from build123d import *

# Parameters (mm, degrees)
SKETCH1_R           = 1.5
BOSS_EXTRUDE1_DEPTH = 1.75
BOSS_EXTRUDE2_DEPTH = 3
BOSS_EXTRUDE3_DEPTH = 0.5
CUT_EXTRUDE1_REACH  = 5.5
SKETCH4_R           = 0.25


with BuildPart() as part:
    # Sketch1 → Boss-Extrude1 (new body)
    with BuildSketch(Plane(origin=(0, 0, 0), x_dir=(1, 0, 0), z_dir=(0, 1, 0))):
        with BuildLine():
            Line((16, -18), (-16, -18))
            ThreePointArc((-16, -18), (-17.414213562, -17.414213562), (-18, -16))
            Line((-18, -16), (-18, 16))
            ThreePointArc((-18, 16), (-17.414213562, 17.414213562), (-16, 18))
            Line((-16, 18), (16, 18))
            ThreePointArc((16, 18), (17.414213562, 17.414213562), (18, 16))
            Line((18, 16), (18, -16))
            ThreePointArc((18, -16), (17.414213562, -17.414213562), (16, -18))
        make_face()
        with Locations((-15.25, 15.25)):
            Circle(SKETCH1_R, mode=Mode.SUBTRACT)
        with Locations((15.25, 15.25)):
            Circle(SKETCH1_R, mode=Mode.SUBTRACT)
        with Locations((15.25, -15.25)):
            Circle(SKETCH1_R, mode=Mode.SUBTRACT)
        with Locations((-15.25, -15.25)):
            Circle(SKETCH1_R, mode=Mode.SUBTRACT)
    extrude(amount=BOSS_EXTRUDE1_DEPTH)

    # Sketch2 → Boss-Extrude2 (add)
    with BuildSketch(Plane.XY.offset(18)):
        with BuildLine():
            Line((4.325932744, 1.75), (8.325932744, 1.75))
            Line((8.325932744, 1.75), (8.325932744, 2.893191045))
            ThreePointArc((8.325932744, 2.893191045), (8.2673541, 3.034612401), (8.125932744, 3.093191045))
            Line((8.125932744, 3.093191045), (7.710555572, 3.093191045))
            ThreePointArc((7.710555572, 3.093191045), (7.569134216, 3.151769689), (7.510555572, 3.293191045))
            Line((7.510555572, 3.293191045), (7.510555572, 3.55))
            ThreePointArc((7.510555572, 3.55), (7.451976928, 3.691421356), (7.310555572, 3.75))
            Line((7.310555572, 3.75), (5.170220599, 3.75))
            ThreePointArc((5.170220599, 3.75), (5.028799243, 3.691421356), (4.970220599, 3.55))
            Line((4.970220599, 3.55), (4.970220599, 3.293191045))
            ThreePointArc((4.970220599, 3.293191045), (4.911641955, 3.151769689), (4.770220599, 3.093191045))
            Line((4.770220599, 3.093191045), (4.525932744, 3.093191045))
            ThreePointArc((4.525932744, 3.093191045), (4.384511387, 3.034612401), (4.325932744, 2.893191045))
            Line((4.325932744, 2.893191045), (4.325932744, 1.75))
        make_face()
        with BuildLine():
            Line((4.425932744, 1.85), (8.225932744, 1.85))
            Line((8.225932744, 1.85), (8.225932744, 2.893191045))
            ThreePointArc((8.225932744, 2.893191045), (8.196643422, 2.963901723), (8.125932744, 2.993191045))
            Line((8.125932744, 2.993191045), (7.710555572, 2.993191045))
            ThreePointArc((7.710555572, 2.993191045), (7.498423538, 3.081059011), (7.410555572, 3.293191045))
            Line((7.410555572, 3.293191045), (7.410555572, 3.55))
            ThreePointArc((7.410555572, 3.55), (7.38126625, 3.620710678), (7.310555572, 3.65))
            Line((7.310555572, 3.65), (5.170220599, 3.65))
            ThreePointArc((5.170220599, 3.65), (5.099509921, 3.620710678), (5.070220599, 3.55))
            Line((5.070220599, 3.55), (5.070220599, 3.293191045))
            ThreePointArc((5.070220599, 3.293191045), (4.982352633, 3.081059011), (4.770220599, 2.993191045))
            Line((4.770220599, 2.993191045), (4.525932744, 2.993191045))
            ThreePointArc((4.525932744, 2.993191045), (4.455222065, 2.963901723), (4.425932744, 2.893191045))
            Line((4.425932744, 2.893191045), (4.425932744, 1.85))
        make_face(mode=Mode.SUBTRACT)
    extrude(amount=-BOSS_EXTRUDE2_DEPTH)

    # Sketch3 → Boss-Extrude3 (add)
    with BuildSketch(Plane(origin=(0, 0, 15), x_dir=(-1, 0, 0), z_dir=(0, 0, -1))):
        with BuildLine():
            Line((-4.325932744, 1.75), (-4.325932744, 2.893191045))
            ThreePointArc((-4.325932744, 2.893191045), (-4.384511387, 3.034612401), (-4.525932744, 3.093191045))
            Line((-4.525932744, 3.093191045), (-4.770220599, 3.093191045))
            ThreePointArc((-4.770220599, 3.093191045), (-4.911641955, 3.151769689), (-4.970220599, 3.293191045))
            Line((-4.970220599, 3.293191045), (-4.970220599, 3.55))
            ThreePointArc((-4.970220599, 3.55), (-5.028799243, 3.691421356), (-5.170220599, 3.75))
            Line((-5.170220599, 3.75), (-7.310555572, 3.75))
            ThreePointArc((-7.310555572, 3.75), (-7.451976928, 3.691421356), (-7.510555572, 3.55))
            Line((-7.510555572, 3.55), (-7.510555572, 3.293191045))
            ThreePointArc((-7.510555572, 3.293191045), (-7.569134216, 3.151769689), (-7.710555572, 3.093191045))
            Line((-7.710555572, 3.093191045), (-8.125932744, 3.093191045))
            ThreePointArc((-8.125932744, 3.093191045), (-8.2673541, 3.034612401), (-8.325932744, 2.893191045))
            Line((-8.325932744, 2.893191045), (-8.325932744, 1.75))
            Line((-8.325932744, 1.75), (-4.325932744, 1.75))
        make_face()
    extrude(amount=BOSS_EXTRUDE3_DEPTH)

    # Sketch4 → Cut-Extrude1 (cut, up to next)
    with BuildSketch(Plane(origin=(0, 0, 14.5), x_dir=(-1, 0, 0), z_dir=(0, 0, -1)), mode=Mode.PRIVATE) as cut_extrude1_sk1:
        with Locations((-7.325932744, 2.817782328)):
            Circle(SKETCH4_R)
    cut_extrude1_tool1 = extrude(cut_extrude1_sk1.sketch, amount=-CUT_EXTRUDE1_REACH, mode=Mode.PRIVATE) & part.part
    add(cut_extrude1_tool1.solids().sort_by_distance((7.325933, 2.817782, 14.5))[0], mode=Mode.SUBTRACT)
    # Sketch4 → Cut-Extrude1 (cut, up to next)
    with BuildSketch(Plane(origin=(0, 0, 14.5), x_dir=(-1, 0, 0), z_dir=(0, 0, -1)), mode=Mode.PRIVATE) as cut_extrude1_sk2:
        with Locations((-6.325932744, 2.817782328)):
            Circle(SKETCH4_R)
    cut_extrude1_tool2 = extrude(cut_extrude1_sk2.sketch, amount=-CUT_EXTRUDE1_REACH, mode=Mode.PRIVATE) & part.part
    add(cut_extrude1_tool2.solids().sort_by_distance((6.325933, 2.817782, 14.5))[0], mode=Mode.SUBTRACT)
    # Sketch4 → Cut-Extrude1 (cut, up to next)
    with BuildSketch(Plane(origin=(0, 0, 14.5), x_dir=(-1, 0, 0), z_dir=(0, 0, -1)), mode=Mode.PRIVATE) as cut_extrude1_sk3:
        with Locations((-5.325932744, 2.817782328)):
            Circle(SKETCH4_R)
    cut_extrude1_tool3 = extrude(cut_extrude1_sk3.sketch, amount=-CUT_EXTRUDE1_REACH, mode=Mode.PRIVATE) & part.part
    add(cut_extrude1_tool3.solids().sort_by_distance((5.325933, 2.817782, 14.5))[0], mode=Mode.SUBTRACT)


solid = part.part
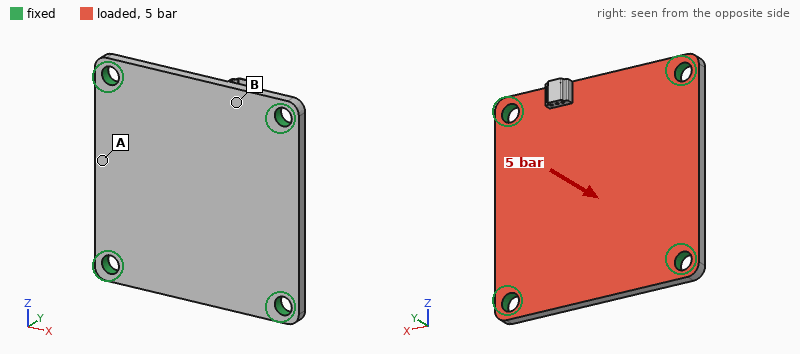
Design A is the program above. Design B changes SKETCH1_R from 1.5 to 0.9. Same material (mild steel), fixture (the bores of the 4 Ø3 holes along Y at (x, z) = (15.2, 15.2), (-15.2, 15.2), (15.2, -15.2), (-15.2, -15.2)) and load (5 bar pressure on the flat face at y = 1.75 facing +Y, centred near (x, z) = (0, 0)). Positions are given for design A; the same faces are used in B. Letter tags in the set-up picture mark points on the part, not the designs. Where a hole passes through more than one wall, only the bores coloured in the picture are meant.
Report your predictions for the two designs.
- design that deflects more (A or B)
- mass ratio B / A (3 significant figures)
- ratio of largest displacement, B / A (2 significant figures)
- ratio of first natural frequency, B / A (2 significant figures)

B
1.01
1.2
0.90
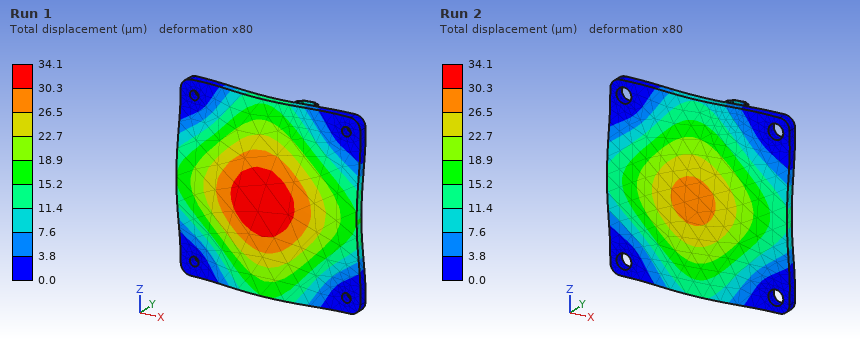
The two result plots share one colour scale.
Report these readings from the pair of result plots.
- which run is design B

Run 1
